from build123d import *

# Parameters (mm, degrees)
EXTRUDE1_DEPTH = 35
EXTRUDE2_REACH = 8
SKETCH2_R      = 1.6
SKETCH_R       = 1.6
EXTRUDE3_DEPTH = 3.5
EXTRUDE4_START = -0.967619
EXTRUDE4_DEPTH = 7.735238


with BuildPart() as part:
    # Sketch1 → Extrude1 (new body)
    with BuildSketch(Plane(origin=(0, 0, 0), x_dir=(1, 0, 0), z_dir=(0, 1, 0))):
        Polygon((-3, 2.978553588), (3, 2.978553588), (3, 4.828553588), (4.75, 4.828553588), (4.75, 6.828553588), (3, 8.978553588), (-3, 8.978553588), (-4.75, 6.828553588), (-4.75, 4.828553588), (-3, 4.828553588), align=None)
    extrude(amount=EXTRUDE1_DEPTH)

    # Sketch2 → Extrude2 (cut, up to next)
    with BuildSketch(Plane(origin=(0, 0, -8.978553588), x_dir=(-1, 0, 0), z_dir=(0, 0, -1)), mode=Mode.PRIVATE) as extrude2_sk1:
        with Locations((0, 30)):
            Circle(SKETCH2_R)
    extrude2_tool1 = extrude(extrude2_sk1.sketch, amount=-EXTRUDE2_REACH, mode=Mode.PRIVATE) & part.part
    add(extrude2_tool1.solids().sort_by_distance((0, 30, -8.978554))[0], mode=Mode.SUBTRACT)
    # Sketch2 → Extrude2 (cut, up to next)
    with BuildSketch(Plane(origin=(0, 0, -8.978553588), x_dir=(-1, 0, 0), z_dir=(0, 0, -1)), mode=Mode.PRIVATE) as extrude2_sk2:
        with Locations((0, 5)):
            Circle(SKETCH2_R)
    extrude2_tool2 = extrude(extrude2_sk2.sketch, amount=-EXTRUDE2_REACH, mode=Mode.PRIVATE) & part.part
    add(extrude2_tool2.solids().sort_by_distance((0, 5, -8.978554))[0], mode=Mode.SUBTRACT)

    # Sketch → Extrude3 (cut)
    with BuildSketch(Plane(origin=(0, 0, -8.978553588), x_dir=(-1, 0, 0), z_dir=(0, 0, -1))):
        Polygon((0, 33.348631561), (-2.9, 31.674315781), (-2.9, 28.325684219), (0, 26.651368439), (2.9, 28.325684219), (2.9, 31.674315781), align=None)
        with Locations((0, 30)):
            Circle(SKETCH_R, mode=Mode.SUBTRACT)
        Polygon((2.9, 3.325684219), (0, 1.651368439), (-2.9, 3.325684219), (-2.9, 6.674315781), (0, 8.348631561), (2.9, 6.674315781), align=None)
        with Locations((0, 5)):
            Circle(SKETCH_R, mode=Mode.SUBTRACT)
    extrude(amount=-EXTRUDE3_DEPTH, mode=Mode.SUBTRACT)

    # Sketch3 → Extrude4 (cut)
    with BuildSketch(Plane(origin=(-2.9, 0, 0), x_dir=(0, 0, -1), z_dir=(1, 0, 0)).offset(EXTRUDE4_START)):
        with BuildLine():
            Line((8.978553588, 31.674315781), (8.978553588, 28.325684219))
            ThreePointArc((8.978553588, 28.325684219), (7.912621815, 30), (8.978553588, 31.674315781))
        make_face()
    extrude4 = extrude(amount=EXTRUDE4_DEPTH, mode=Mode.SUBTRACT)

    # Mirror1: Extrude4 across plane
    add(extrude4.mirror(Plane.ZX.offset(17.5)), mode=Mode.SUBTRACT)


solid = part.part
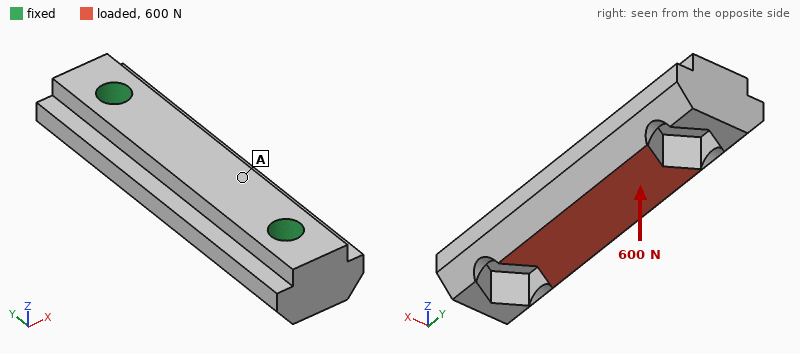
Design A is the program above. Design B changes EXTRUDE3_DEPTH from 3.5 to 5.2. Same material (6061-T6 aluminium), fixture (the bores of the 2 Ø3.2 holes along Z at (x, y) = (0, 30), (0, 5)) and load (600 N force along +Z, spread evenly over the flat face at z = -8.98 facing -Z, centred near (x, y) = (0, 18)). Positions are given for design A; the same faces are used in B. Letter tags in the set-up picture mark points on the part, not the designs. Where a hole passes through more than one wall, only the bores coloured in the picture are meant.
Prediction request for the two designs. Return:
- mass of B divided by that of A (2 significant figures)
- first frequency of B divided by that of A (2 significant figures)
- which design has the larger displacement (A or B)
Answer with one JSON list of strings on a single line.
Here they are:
["0.95", "0.41", "B"]
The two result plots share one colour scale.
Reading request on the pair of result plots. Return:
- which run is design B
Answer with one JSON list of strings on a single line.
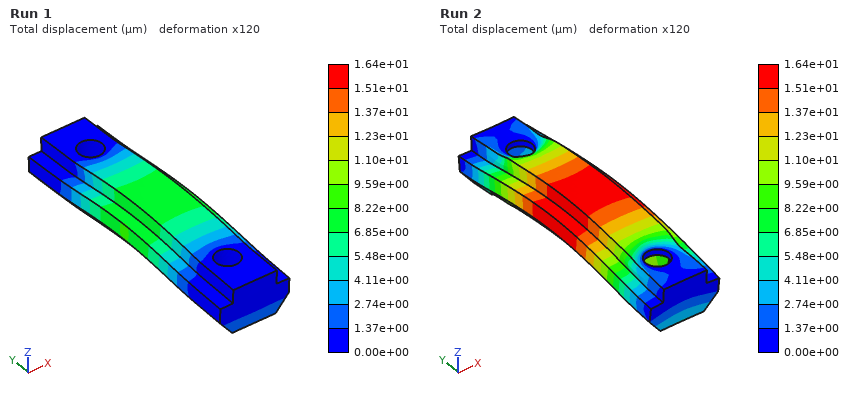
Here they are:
["Run 2"]
